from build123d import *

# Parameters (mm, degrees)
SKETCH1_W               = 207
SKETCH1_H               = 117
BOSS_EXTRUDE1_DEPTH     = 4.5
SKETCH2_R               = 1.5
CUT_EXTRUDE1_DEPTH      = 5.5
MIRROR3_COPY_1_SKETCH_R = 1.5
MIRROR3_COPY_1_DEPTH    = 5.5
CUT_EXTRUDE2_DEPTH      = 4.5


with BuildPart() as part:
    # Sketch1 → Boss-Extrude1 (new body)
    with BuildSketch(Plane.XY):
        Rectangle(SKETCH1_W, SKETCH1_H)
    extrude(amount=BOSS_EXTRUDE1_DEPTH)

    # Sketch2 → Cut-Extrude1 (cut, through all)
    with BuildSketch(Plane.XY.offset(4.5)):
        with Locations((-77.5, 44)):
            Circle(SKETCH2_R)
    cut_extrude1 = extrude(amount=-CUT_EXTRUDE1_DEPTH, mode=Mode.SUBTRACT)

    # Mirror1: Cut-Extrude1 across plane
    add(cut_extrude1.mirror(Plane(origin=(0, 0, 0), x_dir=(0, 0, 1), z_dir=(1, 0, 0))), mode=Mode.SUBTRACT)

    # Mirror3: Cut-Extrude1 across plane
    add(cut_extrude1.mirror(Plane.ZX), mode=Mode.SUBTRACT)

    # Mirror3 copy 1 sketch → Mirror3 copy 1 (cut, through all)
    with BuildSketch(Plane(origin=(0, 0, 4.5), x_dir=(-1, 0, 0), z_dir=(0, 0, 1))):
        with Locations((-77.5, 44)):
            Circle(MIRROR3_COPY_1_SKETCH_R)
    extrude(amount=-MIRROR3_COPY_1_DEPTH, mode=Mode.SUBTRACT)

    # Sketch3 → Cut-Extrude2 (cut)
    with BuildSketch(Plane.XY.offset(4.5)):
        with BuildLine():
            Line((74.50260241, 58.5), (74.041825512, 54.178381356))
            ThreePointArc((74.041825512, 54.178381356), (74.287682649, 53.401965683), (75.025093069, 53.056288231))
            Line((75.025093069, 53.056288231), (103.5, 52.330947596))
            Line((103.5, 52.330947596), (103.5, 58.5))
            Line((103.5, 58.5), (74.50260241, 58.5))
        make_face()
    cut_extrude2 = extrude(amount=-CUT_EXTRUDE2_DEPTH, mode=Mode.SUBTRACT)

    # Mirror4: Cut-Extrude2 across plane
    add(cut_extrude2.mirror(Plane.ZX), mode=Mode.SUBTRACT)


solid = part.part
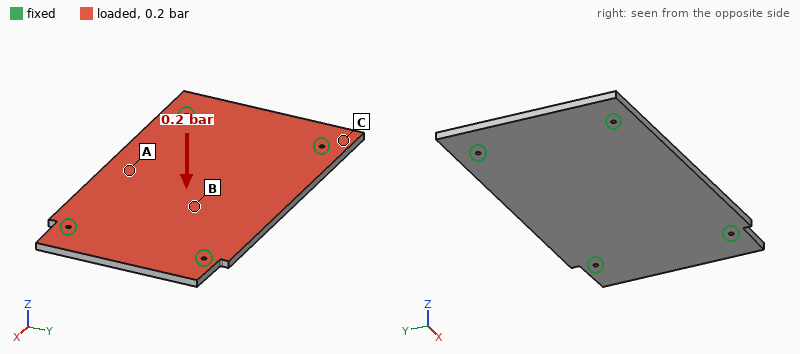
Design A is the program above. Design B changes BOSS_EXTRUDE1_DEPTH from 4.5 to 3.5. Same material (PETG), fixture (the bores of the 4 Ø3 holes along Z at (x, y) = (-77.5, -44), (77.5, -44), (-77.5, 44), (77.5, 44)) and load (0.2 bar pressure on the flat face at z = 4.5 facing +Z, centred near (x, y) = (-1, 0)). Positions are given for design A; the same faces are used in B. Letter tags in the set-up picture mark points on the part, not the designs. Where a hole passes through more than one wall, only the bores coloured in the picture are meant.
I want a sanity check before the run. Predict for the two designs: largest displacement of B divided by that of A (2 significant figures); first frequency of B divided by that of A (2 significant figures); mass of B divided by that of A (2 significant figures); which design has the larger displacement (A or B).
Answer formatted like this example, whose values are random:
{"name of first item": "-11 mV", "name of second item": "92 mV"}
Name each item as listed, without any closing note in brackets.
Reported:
{"largest displacement of B divided by that of A": "2.0", "first frequency of B divided by that of A": "0.79", "mass of B divided by that of A": "0.78", "which design has the larger displacement": "B"}
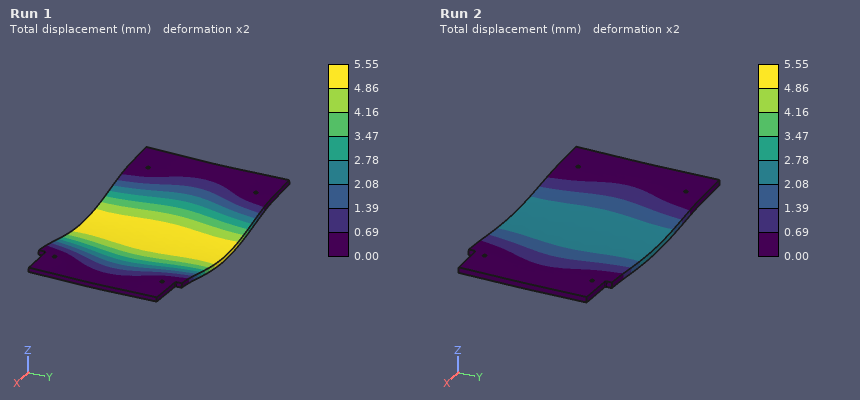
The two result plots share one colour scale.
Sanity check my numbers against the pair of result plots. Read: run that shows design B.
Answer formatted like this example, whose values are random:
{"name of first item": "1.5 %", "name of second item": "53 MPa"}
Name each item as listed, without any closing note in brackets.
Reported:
{"run that shows design B": "Run 1"}
